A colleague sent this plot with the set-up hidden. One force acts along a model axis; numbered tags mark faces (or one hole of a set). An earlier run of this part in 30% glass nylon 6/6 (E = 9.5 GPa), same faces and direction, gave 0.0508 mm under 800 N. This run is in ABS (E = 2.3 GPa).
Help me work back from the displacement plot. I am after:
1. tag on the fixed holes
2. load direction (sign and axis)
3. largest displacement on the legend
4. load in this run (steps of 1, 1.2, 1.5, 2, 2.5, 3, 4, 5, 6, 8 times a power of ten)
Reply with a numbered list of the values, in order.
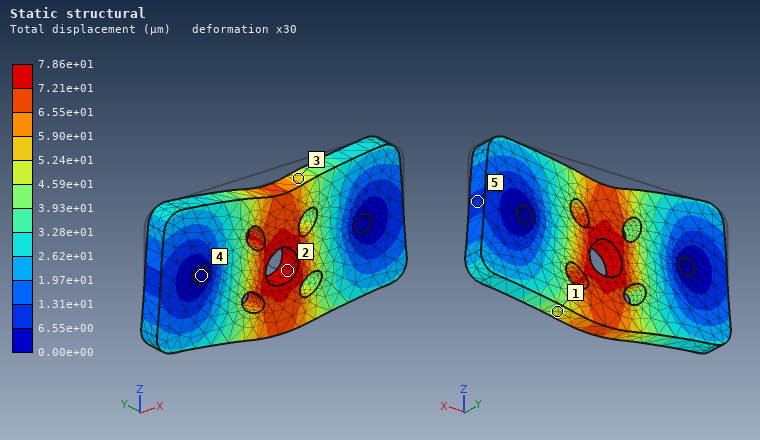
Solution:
1. 4
2. -Z
3. 7.86e+01 µm
4. 300 N
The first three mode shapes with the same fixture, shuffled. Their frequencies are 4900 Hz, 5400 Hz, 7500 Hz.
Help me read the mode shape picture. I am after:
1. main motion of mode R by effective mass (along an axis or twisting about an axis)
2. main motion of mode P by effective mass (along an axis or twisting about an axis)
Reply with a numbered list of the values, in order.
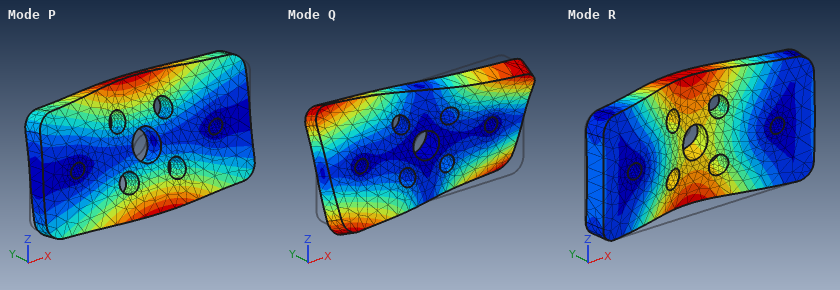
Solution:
1. along Y
2. twisting about X
